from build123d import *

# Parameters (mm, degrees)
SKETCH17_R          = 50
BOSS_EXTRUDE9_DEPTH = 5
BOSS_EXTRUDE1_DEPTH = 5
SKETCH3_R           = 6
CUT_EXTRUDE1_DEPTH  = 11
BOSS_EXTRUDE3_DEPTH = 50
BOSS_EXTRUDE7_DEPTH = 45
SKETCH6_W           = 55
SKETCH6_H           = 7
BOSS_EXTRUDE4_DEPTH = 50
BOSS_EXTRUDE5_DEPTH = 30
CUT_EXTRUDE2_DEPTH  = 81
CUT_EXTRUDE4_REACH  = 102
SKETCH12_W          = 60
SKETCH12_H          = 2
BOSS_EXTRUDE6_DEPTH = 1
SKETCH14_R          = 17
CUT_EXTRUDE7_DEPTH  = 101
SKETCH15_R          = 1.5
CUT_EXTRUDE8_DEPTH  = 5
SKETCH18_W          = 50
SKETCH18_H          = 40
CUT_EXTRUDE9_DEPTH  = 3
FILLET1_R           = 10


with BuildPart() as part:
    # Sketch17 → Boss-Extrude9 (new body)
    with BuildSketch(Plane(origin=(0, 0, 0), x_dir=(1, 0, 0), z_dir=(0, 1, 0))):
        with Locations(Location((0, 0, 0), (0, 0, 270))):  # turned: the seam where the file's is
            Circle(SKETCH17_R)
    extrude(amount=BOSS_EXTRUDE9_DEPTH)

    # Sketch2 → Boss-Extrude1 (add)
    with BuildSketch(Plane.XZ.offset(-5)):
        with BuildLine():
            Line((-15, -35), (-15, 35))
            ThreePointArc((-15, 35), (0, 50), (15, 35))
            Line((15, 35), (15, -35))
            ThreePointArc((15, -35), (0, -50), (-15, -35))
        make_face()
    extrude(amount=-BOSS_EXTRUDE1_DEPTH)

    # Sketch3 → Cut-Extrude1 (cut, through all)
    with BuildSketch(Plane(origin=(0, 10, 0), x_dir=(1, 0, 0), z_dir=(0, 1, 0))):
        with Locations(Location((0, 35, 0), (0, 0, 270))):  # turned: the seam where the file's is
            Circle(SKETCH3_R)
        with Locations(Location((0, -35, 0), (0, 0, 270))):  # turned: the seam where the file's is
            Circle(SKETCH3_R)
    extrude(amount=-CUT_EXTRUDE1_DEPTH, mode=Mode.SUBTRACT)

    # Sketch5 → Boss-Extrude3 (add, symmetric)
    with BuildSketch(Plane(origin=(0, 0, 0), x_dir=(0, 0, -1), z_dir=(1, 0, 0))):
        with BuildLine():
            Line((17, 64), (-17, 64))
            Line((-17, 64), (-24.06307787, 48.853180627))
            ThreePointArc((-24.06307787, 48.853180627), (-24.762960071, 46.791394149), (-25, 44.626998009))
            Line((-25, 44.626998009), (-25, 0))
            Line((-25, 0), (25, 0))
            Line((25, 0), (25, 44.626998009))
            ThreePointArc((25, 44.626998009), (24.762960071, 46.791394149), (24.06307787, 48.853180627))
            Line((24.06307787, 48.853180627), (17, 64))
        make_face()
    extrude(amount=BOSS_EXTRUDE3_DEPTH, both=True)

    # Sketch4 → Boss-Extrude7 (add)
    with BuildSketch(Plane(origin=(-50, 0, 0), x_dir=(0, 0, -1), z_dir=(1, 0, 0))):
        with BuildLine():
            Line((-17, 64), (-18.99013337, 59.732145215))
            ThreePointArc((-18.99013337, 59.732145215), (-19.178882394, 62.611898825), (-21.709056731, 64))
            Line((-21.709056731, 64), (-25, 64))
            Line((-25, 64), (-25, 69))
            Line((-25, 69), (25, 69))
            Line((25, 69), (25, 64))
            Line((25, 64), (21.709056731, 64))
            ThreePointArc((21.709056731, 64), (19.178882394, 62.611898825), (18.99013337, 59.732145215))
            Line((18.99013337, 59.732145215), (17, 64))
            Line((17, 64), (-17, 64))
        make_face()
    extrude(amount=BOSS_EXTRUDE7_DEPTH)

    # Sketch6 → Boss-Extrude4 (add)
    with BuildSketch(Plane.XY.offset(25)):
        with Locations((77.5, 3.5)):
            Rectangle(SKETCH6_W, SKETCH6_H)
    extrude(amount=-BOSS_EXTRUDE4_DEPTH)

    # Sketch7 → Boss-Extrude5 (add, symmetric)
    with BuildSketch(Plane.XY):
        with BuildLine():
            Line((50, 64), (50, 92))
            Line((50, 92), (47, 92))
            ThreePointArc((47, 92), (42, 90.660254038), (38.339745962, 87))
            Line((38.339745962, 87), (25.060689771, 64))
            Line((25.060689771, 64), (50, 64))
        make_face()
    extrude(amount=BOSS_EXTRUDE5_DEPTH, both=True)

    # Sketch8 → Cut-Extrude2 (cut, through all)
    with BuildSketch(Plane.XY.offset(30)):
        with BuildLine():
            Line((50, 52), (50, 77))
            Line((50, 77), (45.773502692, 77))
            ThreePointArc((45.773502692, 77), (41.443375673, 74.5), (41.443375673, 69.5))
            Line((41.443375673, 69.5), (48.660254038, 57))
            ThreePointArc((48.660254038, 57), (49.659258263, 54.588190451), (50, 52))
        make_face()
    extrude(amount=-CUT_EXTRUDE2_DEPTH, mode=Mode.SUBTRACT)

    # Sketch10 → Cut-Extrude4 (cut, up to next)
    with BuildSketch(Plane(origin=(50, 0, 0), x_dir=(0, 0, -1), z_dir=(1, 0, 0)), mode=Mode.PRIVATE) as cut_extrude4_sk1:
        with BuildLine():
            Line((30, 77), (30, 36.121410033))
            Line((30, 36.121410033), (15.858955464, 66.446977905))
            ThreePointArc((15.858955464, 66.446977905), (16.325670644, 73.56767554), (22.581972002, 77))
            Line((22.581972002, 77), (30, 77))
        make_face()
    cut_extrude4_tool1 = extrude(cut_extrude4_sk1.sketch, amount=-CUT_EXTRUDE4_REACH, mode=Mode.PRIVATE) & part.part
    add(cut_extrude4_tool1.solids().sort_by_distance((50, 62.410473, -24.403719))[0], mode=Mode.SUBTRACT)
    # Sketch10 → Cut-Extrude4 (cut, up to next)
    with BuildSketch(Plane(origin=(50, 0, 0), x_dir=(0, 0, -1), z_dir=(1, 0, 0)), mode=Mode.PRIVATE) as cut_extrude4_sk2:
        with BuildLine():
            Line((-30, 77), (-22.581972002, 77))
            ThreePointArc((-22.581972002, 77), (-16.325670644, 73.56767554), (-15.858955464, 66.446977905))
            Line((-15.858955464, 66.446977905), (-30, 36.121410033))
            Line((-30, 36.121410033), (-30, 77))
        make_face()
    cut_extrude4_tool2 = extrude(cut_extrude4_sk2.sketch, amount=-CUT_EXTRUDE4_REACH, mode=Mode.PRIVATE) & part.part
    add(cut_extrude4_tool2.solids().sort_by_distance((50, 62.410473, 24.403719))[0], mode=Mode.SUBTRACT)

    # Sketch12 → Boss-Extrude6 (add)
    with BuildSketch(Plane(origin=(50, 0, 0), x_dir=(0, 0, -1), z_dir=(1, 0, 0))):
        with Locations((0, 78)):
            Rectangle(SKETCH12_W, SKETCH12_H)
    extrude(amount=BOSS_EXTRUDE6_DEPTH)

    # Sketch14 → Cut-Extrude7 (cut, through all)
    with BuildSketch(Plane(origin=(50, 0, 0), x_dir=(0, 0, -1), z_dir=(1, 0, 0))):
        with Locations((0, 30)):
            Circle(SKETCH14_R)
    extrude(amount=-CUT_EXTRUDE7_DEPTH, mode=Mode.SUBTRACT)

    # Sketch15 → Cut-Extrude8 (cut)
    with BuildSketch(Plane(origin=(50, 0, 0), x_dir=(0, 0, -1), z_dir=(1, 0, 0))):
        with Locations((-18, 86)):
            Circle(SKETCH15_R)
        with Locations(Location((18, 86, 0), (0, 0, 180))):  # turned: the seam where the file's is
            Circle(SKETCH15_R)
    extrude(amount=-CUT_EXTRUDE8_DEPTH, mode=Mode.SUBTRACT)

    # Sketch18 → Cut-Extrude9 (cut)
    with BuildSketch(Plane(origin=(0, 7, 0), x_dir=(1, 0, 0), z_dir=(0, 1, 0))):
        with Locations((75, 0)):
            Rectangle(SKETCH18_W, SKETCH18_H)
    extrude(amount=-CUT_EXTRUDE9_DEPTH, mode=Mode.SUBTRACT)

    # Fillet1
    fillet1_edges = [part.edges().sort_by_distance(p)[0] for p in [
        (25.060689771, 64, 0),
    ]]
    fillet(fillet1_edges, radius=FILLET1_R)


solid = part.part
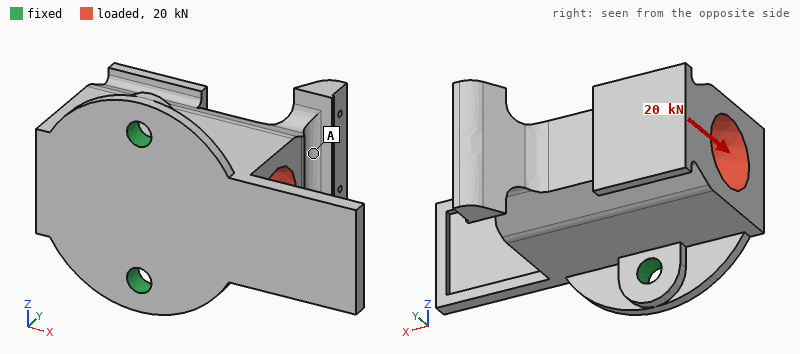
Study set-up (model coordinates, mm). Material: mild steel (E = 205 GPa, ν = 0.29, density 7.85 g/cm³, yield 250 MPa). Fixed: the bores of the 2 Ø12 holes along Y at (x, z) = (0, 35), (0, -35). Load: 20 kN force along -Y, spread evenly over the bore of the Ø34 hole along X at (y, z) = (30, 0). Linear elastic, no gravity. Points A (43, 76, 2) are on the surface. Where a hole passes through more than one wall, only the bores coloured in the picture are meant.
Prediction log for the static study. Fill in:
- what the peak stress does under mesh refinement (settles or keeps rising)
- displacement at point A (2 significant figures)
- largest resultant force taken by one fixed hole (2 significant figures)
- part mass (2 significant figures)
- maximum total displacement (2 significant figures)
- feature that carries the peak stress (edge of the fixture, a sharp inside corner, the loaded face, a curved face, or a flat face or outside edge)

keeps rising
11 µm
11 kN
2.2 kg
17 µm
edge of the fixture
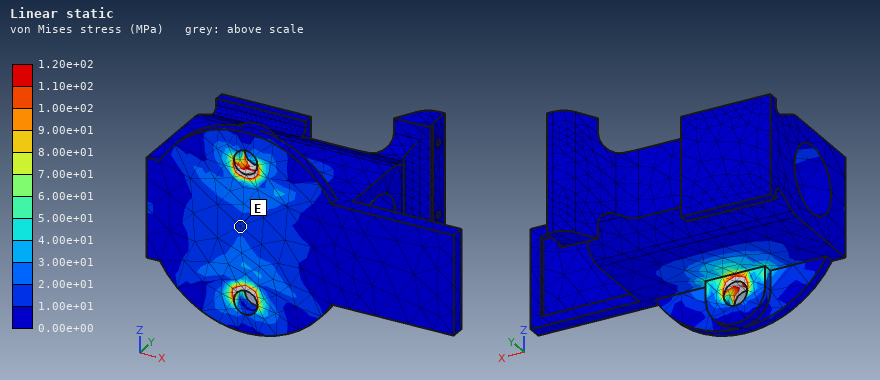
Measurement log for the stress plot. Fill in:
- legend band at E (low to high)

1.00e+01 to 2.00e+01 MPa
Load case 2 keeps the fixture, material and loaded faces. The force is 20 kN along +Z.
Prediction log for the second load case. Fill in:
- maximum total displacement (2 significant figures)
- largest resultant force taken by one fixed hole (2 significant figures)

38 µm
13 kN
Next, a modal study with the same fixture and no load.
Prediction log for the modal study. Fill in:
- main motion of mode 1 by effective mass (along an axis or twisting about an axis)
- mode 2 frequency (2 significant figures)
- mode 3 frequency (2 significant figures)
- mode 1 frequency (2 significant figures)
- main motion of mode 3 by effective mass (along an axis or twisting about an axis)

along X
1400 Hz
2700 Hz
940 Hz
along Z
